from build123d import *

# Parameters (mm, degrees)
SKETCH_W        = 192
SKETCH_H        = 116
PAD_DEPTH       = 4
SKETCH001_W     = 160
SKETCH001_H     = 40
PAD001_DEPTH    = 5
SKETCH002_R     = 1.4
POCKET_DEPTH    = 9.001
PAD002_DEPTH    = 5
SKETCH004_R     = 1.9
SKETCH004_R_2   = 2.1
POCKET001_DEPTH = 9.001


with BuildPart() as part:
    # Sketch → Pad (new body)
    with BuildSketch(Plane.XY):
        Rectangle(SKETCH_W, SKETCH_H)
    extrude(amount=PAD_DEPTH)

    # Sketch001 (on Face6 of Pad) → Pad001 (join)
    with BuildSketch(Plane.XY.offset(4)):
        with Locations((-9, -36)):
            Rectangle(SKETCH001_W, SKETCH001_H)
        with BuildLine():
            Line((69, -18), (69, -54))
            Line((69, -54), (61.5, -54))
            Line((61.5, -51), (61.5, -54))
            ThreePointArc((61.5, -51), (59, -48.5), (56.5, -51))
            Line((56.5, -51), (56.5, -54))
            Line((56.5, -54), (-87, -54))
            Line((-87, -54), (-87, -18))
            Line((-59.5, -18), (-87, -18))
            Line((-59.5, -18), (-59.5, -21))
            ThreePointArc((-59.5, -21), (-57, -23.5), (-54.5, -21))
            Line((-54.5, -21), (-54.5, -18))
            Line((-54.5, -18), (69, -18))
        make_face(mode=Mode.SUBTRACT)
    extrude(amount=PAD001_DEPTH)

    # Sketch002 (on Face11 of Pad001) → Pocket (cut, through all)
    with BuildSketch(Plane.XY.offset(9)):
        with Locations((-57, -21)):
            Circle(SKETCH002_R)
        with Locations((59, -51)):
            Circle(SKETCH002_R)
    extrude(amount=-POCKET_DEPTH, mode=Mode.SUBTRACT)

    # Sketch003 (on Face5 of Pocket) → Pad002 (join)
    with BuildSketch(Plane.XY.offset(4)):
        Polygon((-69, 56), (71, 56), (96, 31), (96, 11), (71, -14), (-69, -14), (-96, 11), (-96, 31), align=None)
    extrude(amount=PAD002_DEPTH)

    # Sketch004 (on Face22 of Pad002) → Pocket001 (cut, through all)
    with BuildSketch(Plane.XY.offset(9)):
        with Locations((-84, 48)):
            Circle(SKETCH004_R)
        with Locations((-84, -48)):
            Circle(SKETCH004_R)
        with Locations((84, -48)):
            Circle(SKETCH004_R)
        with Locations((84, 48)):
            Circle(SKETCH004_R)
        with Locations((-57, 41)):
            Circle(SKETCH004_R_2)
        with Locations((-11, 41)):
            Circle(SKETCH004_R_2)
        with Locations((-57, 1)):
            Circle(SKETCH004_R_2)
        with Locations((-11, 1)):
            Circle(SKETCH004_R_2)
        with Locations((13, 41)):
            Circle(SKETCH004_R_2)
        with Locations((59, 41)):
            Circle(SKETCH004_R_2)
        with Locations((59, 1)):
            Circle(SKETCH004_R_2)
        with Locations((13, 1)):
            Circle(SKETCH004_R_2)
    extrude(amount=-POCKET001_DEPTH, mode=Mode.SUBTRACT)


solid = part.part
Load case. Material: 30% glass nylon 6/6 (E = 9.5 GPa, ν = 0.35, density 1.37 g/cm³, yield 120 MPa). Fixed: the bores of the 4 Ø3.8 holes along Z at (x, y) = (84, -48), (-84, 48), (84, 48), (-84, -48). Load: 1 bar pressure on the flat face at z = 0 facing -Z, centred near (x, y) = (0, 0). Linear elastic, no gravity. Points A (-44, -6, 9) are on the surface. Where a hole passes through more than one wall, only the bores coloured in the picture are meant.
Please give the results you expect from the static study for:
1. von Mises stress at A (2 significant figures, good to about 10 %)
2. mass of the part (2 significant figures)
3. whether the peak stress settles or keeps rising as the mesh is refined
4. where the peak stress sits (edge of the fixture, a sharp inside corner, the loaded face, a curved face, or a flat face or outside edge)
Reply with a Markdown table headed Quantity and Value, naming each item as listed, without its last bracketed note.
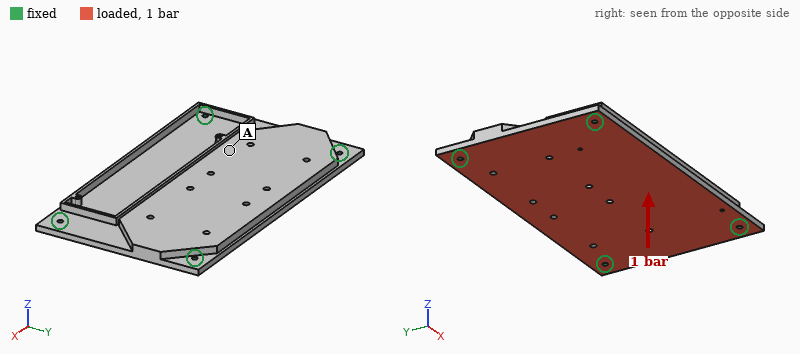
| Quantity | Value |
|---|---|
| von Mises stress at A | 15 MPa |
| mass of the part | 210 g |
| whether the peak stress settles or keeps rising as the mesh is refined | keeps rising |
| where the peak stress sits | edge of the fixture |
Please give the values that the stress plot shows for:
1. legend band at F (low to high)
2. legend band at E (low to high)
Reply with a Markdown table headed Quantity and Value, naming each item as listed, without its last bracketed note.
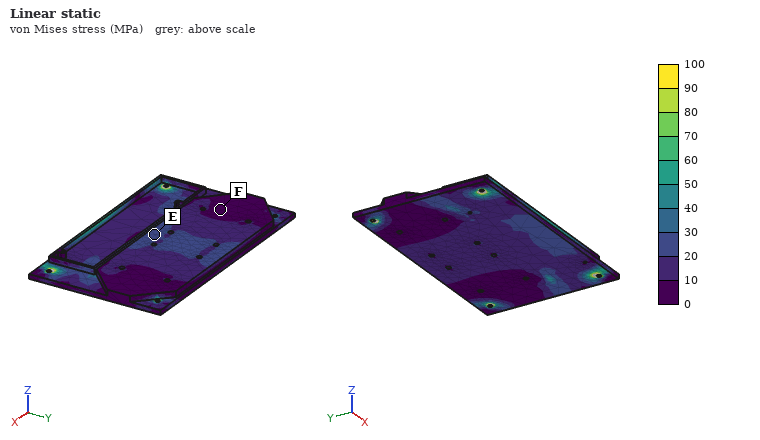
| Quantity | Value |
|---|---|
| legend band at F | 0 to 10 MPa |
| legend band at E | 20 to 30 MPa |
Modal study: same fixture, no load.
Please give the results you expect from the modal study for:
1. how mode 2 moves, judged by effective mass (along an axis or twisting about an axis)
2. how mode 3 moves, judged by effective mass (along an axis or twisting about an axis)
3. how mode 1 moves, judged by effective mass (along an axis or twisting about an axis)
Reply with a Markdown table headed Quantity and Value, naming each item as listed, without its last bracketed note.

| Quantity | Value |
|---|---|
| how mode 2 moves, judged by effective mass | twisting about X |
| how mode 3 moves, judged by effective mass | twisting about Y |
| how mode 1 moves, judged by effective mass | along Z |
